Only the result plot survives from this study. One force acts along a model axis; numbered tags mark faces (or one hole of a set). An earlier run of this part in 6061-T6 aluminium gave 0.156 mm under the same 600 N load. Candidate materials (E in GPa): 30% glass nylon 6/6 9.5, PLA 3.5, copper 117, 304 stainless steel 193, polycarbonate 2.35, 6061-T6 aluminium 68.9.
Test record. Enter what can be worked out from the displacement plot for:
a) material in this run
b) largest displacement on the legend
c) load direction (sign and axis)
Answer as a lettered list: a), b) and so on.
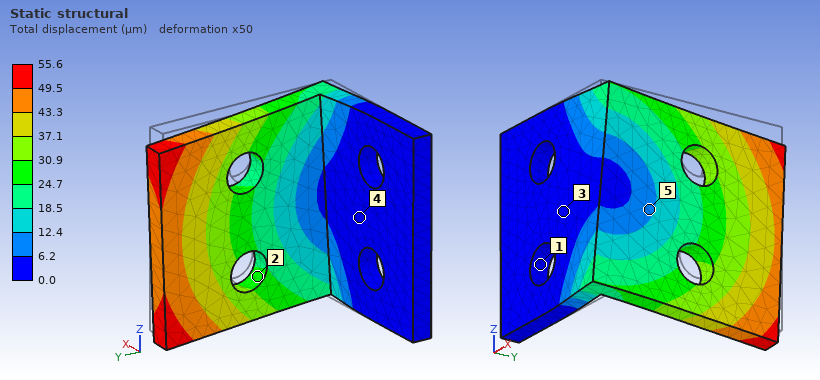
a) 304 stainless steel
b) 55.6 µm
c) -Z
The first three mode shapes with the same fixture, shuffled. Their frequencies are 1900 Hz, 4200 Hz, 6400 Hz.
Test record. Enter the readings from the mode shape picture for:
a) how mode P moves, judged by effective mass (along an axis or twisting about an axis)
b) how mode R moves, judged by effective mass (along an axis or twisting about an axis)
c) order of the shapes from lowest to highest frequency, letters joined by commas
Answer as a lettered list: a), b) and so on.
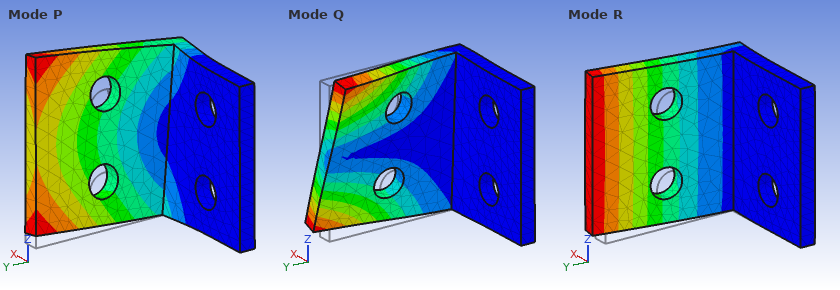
a) along Z
b) along X
c) R, P, Q
